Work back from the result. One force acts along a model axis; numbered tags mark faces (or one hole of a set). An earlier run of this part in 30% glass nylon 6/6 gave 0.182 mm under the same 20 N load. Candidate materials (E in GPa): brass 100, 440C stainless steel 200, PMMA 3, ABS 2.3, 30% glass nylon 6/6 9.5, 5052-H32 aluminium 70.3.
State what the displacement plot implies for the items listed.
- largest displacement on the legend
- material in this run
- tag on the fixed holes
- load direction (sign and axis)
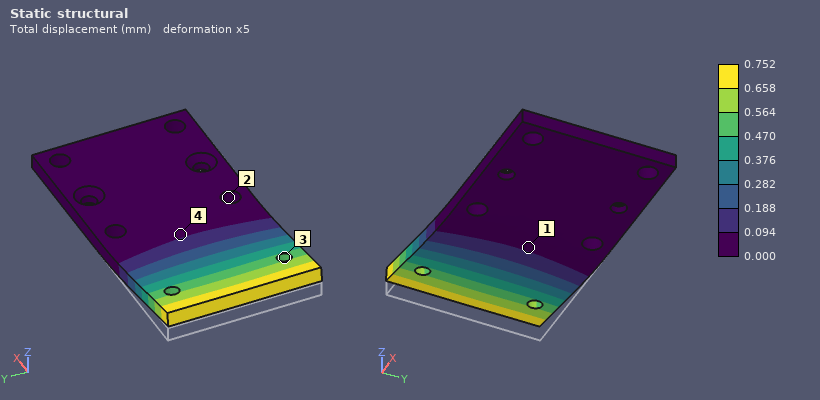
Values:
0.752 mm
ABS
2
+Z
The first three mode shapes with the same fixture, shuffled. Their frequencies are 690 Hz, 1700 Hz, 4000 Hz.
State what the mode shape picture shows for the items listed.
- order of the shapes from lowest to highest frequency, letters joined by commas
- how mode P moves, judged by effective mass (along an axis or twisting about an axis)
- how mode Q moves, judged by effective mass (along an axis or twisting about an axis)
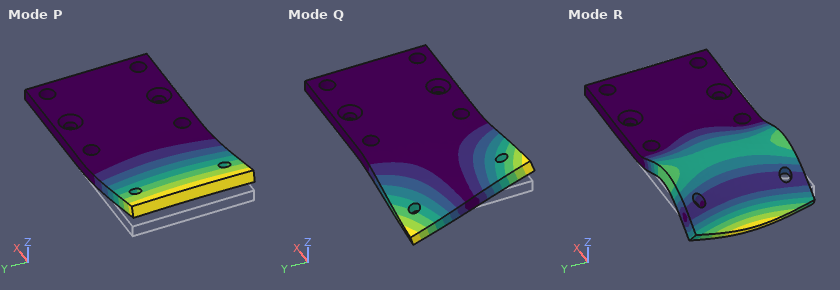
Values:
P, Q, R
along Z
twisting about X
